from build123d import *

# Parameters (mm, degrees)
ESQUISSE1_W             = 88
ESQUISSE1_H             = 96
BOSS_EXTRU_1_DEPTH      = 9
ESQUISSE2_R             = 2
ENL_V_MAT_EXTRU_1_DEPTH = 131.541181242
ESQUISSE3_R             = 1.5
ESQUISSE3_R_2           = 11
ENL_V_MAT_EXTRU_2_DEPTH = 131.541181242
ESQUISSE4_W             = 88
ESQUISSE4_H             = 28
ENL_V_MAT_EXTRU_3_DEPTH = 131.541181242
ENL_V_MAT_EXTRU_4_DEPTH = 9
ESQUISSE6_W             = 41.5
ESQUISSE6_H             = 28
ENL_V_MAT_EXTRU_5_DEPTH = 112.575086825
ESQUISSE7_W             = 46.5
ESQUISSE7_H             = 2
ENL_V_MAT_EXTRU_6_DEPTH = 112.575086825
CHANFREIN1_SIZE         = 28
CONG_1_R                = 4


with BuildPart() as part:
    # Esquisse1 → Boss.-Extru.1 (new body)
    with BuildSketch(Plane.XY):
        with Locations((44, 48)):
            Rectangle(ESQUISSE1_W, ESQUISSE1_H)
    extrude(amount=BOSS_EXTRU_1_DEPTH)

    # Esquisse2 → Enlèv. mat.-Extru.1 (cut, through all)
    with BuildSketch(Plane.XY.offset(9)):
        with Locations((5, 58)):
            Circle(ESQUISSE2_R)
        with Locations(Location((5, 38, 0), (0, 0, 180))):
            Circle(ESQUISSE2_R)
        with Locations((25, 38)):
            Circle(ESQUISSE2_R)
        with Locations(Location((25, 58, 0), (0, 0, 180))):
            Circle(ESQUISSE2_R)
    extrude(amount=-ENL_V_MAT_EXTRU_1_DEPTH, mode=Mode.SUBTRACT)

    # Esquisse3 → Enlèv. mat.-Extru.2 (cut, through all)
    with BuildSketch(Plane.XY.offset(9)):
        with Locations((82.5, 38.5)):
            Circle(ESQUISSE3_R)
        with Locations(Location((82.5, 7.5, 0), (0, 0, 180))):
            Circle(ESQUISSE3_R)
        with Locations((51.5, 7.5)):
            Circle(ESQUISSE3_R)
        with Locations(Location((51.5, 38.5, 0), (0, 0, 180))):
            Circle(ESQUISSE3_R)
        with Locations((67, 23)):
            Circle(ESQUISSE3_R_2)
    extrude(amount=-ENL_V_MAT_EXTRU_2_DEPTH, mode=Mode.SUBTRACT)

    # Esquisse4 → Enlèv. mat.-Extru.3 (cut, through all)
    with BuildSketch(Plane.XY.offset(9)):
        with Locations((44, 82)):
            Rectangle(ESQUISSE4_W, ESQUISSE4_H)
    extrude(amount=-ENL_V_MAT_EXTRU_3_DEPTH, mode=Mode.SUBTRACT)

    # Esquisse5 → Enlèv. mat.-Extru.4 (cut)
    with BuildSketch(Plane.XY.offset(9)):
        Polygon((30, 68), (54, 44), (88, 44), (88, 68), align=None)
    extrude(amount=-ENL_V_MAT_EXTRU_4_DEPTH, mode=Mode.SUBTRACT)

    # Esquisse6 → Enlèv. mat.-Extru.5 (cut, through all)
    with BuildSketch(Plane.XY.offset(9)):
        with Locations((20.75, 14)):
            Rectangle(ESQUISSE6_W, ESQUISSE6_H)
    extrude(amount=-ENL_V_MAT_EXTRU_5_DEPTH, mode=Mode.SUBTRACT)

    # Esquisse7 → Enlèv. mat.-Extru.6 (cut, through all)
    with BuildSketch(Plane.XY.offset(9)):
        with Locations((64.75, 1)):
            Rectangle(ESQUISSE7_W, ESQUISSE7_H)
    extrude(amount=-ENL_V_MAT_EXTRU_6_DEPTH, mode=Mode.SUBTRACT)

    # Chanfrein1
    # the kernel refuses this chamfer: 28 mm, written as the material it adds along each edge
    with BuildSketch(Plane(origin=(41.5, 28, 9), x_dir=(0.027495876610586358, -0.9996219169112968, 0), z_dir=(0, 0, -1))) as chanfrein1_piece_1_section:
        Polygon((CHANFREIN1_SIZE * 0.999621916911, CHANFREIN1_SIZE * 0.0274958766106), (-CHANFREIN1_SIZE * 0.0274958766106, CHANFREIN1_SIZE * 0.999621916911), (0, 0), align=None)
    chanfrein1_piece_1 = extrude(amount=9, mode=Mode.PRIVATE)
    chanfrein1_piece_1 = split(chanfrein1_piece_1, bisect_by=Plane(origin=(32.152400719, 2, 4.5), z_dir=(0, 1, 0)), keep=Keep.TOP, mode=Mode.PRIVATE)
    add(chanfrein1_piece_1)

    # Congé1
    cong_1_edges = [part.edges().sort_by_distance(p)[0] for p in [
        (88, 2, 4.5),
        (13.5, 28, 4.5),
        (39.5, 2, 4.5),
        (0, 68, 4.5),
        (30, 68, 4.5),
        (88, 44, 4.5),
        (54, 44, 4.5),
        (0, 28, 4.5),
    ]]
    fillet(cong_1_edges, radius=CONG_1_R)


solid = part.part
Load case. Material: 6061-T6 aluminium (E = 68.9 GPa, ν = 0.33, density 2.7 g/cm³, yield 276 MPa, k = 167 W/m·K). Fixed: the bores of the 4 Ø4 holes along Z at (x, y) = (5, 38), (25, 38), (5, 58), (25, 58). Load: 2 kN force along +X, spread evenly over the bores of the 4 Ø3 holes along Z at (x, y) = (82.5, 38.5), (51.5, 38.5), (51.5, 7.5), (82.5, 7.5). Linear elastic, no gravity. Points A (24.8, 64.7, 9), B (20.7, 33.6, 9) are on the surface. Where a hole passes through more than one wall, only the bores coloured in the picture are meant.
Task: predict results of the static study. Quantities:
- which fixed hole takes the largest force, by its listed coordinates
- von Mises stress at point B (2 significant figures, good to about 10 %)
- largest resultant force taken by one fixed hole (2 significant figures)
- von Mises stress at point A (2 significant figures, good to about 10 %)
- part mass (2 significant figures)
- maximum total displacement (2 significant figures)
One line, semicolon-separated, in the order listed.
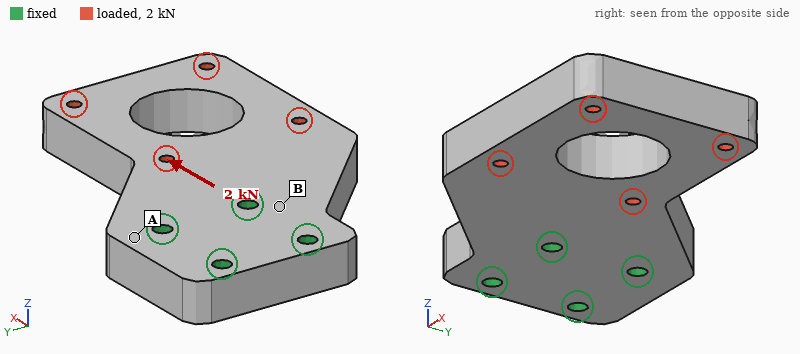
(25, 38); 10 MPa; 1.8 kN; 3.7 MPa; 86 g; 29 µm
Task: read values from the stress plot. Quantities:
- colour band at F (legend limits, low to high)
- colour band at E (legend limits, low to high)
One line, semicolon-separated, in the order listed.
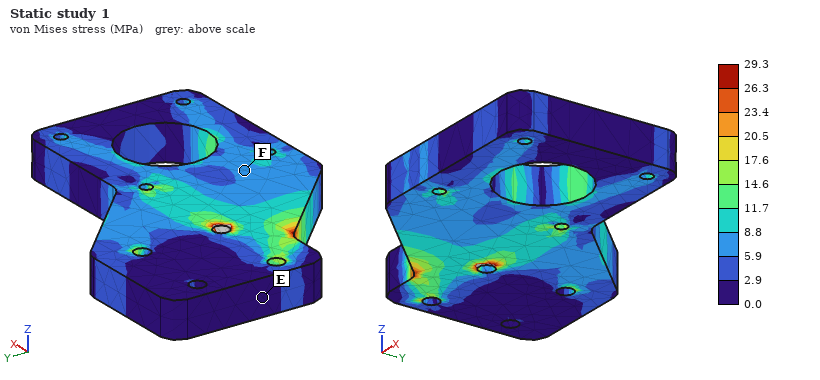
5.9 to 8.8 MPa; 0.0 to 2.9 MPa
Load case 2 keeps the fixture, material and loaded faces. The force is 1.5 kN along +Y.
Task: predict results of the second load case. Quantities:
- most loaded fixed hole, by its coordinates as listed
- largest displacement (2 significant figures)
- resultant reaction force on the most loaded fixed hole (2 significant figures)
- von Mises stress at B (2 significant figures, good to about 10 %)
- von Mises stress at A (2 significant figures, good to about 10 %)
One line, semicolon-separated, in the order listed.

(25, 58); 59 µm; 2.2 kN; 10 MPa; 9.1 MPa
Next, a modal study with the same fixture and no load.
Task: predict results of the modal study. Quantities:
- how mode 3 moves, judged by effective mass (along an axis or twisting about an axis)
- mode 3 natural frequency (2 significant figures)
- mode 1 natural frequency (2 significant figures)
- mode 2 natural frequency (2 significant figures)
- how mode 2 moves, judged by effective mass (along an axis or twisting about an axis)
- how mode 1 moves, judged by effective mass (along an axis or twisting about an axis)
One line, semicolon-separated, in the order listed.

along Y; 4900 Hz; 1700 Hz; 4200 Hz; twisting about X; along Z
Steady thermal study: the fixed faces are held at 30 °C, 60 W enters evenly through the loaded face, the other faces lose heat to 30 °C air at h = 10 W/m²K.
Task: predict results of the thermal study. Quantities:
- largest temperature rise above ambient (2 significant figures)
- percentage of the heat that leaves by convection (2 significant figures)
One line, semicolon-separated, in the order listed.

60 K; 4.1 %
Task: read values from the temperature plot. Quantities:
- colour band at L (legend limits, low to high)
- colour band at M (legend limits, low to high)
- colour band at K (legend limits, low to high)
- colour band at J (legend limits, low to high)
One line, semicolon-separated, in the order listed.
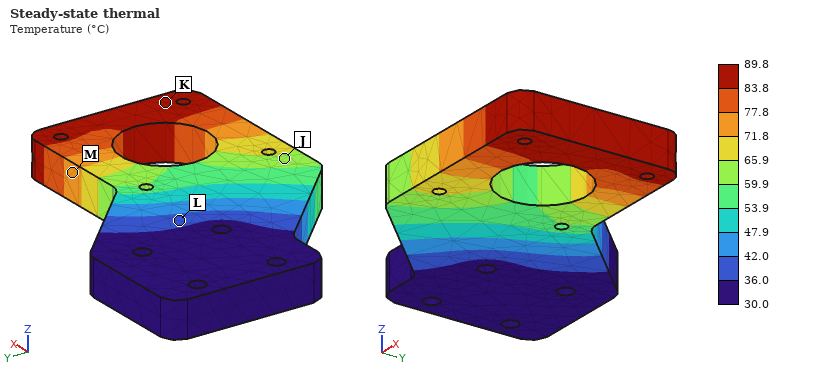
36.0 to 42.0 °C; 71.8 to 77.8 °C; 83.8 to 89.8 °C; 59.9 to 65.9 °C
